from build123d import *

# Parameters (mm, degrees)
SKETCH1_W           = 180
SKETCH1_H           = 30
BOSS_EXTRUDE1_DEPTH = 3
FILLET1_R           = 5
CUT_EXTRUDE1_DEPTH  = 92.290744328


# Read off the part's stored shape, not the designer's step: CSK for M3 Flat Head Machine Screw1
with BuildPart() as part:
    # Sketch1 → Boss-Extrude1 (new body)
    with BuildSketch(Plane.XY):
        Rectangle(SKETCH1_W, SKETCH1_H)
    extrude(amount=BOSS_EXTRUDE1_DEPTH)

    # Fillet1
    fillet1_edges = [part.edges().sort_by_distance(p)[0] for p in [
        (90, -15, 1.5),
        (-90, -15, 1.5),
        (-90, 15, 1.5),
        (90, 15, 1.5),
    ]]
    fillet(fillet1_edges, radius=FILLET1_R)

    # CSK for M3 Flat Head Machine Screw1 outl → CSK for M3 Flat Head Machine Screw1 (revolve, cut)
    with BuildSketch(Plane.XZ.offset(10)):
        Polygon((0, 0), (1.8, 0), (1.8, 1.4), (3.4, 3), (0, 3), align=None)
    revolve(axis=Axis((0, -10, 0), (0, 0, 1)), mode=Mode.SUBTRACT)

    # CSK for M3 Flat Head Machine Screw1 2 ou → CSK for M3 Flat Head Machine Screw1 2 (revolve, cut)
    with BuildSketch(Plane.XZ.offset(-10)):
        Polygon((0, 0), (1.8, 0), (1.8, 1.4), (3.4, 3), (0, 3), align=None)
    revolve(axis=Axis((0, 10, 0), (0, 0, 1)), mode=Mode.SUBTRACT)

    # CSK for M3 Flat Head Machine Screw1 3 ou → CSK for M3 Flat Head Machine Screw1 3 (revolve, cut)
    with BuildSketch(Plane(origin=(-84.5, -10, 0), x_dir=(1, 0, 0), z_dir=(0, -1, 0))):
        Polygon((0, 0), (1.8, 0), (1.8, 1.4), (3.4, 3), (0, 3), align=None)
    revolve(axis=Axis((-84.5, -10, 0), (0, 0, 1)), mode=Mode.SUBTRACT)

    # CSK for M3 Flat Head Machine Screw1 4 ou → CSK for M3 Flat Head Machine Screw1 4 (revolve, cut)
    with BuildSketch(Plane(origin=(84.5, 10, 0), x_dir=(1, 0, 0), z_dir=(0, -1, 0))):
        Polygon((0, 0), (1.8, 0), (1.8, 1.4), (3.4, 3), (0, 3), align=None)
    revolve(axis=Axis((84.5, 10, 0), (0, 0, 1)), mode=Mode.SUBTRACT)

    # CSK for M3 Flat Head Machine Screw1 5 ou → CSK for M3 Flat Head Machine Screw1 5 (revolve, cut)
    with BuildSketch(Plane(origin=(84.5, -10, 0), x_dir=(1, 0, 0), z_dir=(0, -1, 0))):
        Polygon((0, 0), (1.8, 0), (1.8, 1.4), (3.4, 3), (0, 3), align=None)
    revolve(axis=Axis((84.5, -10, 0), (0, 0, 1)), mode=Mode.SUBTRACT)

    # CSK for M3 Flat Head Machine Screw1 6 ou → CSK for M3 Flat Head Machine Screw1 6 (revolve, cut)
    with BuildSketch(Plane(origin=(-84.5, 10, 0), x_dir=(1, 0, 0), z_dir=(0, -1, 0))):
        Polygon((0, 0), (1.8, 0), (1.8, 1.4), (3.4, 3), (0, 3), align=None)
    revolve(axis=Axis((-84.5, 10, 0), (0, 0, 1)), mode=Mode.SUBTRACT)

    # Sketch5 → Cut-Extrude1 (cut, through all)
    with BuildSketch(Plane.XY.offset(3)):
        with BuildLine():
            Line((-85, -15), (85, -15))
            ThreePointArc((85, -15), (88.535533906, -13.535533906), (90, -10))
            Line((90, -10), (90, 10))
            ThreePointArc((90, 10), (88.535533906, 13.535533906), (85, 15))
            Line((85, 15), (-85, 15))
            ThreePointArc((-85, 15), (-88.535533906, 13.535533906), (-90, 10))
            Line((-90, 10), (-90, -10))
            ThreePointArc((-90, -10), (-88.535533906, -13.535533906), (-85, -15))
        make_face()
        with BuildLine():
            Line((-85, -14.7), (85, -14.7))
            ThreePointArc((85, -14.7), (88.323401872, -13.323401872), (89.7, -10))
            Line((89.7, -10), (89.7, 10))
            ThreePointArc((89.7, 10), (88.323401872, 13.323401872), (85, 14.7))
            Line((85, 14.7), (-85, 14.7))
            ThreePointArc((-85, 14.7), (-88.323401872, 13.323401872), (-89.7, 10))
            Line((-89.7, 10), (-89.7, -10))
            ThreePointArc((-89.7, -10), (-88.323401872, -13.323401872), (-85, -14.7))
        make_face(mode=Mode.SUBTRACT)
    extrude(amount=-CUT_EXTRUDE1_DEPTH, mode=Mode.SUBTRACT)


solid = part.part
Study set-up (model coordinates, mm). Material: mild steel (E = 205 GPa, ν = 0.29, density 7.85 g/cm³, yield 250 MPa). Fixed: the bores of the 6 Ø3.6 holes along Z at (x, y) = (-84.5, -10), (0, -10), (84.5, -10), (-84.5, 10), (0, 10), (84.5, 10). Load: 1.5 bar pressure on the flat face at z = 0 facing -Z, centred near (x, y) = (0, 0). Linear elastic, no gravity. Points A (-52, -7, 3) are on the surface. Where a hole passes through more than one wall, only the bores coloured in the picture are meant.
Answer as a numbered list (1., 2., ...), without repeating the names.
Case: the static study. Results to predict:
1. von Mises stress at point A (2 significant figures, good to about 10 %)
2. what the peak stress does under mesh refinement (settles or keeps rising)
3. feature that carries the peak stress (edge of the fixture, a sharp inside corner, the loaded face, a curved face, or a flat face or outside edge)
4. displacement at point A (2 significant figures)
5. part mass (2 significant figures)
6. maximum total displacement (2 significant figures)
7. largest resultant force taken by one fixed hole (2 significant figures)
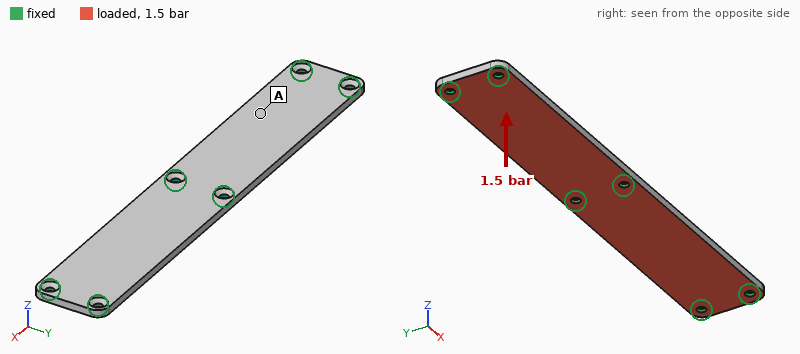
1. 29 MPa
2. keeps rising
3. edge of the fixture
4. 45 µm
5. 120 g
6. 51 µm
7. 220 N
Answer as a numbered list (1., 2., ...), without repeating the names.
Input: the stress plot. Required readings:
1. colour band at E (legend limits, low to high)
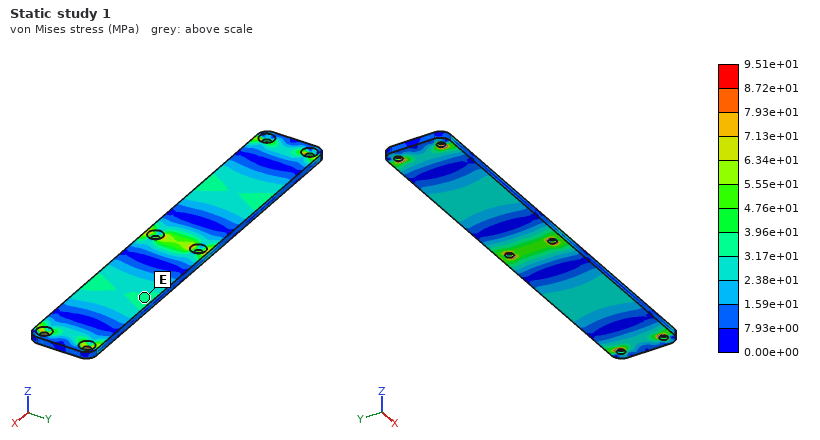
1. 3.17e+01 to 3.96e+01 MPa
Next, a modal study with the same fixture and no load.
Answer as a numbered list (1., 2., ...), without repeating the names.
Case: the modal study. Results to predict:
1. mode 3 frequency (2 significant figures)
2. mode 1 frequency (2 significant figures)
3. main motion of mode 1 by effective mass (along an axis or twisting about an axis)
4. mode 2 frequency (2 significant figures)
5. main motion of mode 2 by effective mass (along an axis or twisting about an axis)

1. 4300 Hz
2. 1900 Hz
3. twisting about Y
4. 2100 Hz
5. along Z
